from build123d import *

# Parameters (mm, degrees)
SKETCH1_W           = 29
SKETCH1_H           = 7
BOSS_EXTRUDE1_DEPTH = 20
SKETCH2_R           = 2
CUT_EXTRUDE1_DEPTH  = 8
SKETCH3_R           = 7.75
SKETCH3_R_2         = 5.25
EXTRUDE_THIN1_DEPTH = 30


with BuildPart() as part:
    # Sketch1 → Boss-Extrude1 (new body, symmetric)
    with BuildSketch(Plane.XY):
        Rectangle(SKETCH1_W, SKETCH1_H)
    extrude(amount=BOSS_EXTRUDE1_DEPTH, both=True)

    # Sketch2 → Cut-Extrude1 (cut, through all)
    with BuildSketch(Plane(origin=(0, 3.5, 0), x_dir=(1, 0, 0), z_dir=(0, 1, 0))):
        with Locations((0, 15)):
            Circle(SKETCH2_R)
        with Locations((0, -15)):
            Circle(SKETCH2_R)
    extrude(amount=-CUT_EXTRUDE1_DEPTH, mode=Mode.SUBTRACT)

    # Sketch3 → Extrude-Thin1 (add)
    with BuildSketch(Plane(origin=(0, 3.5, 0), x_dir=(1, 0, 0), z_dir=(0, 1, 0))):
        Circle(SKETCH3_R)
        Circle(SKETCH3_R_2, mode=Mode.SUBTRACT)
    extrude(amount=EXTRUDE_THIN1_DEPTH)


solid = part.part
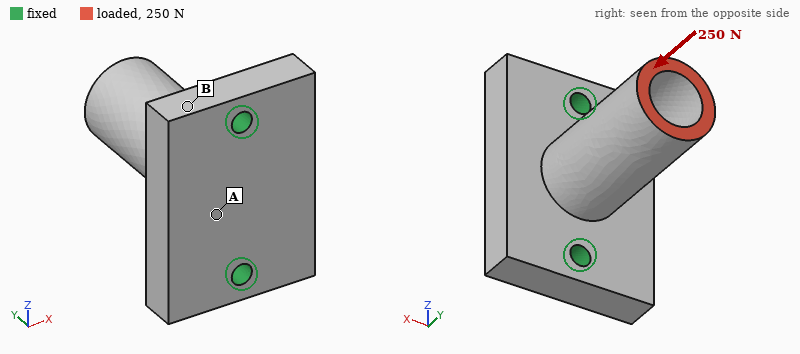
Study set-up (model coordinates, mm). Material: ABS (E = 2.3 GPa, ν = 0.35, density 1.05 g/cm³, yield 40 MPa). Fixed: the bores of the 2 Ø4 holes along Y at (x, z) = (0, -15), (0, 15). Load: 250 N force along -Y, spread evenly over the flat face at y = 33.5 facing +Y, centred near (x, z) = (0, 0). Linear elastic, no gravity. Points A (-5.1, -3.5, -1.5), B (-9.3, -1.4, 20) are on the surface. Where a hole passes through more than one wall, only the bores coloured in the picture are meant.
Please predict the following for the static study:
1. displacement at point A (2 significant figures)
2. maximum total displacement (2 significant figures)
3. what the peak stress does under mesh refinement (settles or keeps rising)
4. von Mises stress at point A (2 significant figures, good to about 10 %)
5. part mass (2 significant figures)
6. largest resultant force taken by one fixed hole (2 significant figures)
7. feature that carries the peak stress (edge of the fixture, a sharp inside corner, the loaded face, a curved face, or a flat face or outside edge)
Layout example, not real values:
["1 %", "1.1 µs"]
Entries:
["28 µm", "59 µm", "keeps rising", "2.0 MPa", "12 g", "130 N", "edge of the fixture"]
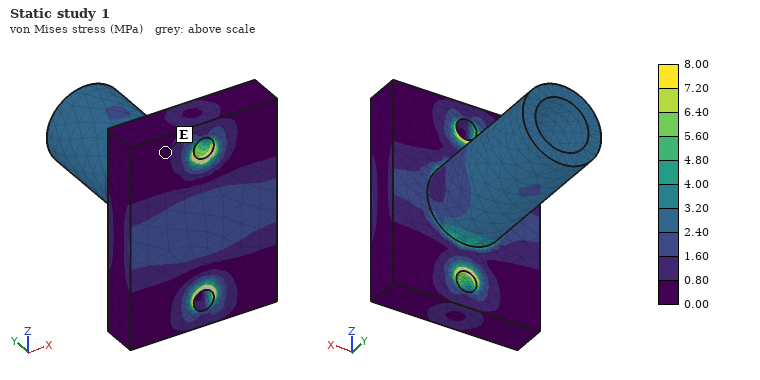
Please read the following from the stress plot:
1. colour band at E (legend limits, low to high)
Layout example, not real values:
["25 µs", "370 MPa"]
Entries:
["0.00 to 0.80 MPa"]
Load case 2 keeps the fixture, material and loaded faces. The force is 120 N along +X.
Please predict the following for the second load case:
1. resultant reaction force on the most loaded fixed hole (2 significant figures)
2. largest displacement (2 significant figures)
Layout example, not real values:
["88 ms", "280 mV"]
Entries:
["60 N", "0.71 mm"]
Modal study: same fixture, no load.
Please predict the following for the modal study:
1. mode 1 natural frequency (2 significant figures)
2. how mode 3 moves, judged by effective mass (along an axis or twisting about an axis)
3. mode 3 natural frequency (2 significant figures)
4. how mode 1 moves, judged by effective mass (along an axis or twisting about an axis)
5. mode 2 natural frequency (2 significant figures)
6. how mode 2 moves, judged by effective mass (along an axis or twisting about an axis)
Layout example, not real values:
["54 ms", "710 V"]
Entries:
["1900 Hz", "along Y", "5200 Hz", "along X", "2800 Hz", "along Z"]
